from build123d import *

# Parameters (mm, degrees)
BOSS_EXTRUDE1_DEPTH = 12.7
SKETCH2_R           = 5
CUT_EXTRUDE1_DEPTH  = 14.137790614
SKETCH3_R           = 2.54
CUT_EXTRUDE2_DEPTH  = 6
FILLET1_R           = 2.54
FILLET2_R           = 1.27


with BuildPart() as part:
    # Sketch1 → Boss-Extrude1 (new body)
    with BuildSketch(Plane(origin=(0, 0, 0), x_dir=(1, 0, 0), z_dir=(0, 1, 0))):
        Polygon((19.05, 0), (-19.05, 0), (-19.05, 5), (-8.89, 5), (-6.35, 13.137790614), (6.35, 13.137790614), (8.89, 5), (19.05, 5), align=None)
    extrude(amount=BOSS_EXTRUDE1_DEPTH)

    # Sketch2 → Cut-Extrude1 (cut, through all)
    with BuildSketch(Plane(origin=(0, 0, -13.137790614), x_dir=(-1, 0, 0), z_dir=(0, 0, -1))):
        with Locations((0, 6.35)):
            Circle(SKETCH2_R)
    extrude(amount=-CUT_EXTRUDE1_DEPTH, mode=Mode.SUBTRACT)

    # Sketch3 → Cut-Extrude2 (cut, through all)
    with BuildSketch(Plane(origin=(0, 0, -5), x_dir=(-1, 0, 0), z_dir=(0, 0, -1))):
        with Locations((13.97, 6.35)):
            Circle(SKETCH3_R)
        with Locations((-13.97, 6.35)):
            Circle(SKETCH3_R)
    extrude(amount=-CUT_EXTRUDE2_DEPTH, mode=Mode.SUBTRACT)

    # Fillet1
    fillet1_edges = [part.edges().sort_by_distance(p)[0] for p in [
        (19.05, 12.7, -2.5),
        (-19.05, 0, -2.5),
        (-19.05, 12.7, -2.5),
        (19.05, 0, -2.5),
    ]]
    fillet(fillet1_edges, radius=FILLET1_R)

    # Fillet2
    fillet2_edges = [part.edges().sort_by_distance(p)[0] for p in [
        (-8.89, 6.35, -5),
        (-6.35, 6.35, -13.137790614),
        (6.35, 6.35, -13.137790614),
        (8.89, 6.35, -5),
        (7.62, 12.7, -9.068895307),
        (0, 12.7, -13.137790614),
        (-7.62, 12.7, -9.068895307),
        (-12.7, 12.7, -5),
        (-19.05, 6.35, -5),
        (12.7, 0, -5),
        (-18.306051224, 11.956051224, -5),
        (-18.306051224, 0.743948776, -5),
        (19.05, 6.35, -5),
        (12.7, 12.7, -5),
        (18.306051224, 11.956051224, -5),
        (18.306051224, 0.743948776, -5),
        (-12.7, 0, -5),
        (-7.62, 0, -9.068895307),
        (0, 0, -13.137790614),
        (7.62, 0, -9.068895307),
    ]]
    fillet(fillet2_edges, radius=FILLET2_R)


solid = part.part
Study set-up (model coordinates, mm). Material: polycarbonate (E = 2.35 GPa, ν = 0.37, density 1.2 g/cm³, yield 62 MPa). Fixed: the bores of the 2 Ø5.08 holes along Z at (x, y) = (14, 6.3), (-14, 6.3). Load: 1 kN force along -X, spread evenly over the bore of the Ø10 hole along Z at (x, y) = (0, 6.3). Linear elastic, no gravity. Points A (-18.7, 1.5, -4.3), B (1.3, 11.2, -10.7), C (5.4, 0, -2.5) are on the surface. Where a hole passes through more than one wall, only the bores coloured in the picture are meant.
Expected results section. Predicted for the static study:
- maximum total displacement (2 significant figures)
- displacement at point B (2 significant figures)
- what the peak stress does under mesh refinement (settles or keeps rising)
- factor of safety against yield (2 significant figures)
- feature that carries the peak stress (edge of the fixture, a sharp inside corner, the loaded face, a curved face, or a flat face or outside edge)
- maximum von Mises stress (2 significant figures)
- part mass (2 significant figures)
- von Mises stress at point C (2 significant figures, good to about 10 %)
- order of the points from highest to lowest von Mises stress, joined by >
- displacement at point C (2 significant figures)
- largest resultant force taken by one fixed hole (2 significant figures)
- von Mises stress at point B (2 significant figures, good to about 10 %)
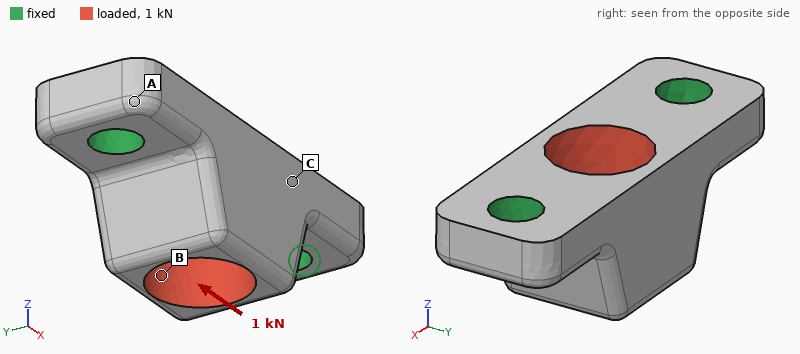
0.11 mm
0.078 mm
settles
1.8
a curved face
34 MPa
3.2 g
5.9 MPa
B > C > A
0.028 mm
530 N
11 MPa
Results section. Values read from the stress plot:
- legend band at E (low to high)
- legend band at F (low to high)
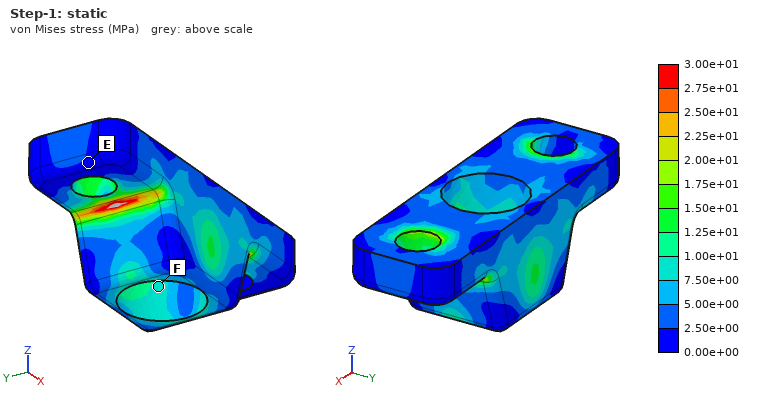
0.00e+00 to 2.50e+00 MPa
7.50e+00 to 1.00e+01 MPa
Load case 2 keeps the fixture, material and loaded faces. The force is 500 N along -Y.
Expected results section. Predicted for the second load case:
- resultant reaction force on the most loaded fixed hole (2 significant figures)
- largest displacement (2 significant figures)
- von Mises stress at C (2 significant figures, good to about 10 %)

250 N
0.25 mm
5.9 MPa
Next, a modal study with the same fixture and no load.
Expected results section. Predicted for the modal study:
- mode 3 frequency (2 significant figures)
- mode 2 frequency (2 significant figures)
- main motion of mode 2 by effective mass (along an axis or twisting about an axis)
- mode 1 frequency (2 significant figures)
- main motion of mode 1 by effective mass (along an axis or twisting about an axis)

11 kHz
9600 Hz
along Z
6300 Hz
along Y
